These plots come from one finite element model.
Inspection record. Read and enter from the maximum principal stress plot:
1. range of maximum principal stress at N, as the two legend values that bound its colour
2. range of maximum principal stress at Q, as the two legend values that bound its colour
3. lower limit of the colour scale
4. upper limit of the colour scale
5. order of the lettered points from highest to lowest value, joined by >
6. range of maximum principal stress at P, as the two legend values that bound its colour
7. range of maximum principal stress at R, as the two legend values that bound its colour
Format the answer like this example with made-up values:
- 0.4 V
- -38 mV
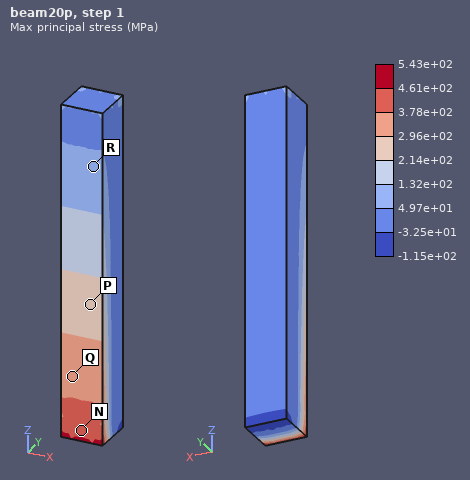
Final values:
- 3.78e+02 to 4.61e+02 MPa
- 2.96e+02 to 3.78e+02 MPa
- -1.15e+02 MPa
- 5.43e+02 MPa
- N > Q > P > R
- 2.14e+02 to 2.96e+02 MPa
- 4.97e+01 to 1.32e+02 MPa
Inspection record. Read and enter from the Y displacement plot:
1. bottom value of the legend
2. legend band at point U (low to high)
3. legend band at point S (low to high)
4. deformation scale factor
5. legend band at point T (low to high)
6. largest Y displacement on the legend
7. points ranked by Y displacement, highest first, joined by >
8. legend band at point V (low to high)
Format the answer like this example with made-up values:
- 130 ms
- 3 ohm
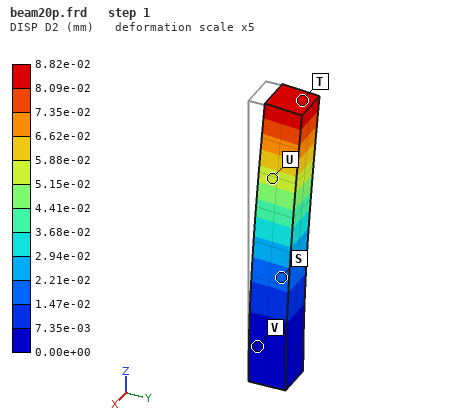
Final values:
- 0.00e+00 mm
- 5.15e-02 to 5.88e-02 mm
- 1.47e-02 to 2.21e-02 mm
- 5
- 8.09e-02 to 8.82e-02 mm
- 8.82e-02 mm
- T > U > S > V
- 0.00e+00 to 7.35e-03 mm
